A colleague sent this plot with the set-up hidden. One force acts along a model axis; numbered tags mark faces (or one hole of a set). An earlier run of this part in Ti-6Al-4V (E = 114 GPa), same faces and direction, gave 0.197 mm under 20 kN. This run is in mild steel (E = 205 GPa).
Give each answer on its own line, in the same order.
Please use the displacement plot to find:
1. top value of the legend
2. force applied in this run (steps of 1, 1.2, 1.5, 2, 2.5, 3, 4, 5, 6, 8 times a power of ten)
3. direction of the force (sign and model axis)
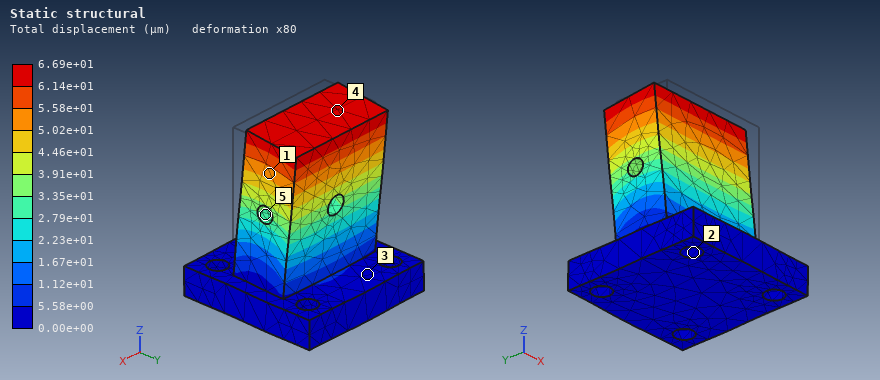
6.69e+01 µm
12 kN
+Y
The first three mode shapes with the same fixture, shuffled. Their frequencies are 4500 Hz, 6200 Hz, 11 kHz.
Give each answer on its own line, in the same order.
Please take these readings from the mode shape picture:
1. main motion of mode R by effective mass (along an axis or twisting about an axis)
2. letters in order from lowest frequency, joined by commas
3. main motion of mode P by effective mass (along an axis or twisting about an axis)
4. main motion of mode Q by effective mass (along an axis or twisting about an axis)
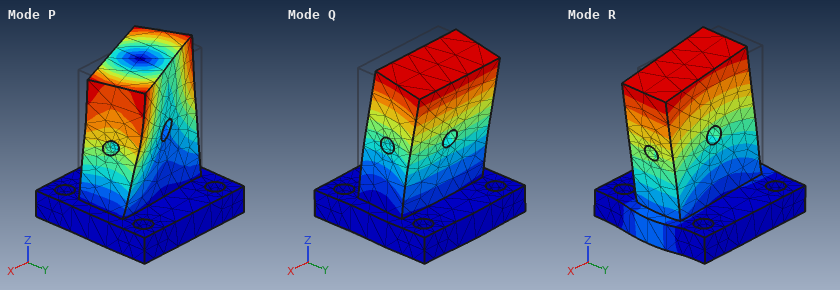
along X
Q, R, P
twisting about Z
along Y
